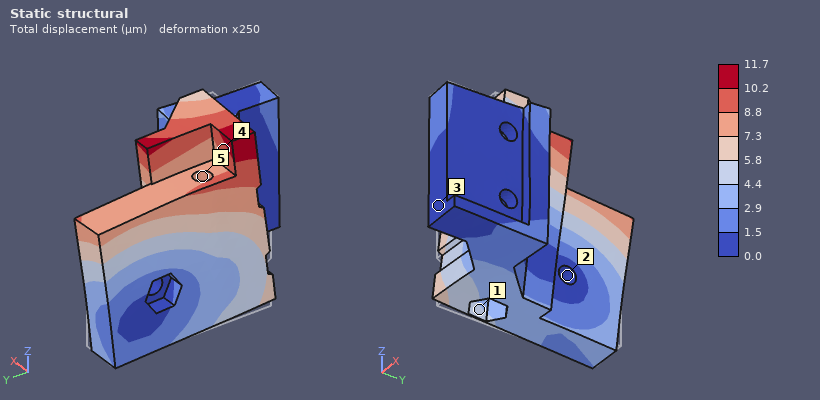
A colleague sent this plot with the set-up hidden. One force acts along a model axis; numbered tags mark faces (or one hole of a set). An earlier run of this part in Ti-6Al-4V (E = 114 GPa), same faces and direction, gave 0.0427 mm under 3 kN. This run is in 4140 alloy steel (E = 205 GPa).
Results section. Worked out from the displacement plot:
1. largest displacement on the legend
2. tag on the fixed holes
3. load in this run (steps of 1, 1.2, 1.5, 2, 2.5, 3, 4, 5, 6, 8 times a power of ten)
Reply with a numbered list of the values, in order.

1. 11.7 µm
2. 2
3. 1.5 kN
